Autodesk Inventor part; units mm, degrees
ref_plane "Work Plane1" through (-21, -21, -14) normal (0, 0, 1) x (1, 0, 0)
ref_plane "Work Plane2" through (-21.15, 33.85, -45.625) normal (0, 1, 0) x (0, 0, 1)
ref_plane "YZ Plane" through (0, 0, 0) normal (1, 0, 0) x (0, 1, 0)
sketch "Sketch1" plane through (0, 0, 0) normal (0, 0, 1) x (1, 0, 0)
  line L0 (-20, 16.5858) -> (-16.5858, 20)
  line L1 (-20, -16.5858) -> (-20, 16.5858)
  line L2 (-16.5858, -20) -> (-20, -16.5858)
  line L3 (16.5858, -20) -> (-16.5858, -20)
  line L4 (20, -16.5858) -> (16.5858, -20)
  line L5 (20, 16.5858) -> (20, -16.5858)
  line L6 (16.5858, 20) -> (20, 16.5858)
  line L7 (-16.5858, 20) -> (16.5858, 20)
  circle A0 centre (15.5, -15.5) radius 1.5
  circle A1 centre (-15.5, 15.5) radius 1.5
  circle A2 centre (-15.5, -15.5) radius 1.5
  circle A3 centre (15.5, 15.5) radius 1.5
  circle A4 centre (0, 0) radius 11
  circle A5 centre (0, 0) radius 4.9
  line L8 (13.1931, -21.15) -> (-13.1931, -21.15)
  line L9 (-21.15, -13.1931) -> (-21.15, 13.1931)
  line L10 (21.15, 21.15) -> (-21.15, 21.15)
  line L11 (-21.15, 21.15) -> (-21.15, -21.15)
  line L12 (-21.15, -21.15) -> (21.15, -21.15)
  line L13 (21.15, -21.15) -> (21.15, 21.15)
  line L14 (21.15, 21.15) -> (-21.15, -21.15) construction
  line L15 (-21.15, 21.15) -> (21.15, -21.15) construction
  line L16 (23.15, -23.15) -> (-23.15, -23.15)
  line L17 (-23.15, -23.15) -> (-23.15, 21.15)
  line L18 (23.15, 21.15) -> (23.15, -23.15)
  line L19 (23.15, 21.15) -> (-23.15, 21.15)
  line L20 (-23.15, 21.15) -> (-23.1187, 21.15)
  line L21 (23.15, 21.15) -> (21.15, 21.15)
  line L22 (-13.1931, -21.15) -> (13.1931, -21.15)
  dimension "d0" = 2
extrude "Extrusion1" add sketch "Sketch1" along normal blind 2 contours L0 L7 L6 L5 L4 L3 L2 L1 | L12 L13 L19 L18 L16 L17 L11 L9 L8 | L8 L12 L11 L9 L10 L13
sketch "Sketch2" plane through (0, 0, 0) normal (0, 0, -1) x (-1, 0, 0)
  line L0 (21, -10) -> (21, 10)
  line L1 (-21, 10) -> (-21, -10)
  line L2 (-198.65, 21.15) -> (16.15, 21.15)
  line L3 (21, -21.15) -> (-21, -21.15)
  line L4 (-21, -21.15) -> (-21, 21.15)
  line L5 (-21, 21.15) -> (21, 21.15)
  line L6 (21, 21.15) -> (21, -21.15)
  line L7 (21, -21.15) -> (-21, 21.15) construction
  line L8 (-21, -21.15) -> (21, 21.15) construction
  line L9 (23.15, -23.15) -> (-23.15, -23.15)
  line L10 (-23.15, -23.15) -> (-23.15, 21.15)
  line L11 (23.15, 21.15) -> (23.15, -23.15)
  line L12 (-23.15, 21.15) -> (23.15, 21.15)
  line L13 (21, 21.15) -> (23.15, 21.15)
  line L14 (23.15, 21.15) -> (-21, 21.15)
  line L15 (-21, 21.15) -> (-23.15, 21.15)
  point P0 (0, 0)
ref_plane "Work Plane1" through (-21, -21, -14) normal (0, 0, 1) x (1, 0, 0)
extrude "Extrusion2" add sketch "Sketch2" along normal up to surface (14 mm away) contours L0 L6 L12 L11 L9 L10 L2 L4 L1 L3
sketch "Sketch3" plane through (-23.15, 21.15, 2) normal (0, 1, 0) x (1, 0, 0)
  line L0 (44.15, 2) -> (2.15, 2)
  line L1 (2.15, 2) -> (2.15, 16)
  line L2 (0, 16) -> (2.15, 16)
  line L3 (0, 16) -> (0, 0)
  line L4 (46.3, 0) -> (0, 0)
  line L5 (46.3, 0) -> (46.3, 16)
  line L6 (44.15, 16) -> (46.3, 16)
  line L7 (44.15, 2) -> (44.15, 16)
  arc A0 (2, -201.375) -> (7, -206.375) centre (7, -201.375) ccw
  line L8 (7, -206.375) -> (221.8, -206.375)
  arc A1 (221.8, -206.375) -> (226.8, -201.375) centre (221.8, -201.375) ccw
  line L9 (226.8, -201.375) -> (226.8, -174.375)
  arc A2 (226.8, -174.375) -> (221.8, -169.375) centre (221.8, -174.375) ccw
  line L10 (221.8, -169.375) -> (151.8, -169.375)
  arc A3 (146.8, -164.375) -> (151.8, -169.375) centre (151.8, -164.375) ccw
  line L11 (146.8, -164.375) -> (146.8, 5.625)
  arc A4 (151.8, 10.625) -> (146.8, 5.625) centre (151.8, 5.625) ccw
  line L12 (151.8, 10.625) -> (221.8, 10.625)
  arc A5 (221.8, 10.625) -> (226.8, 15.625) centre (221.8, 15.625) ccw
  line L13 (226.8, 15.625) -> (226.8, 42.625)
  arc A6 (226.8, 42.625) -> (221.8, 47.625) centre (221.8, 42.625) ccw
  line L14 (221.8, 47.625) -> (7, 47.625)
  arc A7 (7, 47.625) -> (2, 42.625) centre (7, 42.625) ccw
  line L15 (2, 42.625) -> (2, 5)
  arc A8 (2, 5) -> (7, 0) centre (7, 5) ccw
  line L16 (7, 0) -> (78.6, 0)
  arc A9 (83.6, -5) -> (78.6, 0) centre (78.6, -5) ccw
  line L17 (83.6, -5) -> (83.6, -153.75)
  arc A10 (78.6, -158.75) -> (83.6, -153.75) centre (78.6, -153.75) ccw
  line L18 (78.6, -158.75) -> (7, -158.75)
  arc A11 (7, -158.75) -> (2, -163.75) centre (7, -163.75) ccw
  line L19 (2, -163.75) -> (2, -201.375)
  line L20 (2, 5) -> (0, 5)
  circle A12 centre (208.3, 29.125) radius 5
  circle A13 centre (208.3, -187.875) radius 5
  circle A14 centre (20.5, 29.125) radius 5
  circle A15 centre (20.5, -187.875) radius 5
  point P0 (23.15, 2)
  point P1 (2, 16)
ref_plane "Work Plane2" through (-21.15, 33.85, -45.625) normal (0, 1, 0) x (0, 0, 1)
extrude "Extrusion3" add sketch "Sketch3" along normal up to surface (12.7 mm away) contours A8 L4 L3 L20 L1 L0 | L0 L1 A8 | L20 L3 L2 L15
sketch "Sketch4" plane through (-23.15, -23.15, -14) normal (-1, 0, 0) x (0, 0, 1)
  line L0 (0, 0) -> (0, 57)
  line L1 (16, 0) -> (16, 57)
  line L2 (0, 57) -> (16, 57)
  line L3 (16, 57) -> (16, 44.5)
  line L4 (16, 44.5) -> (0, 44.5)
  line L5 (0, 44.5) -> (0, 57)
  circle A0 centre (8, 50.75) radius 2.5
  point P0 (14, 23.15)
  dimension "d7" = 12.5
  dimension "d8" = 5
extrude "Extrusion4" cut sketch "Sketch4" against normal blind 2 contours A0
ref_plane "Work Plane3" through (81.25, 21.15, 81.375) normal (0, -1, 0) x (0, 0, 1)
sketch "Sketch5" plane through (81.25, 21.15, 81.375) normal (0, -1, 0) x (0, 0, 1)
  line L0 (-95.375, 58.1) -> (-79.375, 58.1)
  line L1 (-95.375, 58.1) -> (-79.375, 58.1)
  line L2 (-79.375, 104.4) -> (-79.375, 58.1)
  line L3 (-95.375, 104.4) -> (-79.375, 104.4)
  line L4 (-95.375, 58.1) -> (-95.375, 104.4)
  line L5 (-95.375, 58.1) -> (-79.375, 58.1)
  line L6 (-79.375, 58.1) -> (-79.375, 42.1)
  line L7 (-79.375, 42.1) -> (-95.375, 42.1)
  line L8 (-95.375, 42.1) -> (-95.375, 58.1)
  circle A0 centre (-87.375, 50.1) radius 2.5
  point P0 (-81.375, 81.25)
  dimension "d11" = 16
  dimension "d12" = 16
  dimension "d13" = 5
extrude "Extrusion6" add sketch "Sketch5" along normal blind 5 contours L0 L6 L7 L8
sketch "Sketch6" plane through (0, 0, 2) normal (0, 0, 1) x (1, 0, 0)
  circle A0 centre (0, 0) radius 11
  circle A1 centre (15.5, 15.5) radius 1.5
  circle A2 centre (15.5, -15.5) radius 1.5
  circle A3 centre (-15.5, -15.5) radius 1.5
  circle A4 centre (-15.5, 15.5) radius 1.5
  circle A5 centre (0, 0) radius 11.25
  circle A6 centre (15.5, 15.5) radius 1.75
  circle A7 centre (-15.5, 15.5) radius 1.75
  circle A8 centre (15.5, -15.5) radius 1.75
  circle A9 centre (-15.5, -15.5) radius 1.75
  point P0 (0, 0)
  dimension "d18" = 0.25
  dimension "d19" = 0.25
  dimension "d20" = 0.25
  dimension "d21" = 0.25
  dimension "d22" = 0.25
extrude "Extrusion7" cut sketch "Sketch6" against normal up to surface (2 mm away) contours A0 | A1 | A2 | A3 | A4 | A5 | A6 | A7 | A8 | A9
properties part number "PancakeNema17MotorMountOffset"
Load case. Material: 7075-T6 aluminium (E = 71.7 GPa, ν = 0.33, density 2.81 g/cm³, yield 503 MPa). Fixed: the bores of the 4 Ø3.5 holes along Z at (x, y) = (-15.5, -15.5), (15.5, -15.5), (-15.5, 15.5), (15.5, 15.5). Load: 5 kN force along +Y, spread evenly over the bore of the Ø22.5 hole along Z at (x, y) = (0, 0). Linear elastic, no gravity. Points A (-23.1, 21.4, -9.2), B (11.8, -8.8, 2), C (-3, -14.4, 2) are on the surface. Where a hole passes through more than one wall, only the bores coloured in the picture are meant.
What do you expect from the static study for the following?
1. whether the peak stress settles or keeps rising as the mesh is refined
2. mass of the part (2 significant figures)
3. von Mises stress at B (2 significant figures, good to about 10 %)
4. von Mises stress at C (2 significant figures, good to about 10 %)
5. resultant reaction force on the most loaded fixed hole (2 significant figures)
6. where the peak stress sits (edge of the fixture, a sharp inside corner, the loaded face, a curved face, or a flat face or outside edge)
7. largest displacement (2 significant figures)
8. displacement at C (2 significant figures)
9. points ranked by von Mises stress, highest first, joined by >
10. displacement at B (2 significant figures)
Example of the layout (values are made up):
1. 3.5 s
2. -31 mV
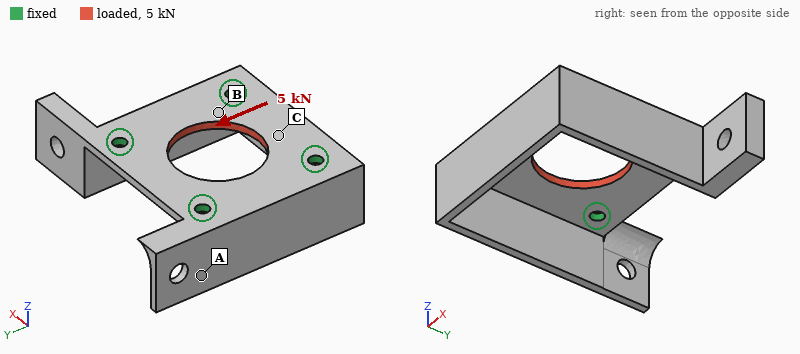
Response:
1. keeps rising
2. 24 g
3. 52 MPa
4. 31 MPa
5. 1.3 kN
6. edge of the fixture
7. 21 µm
8. 14 µm
9. B > C > A
10. 6.3 µm
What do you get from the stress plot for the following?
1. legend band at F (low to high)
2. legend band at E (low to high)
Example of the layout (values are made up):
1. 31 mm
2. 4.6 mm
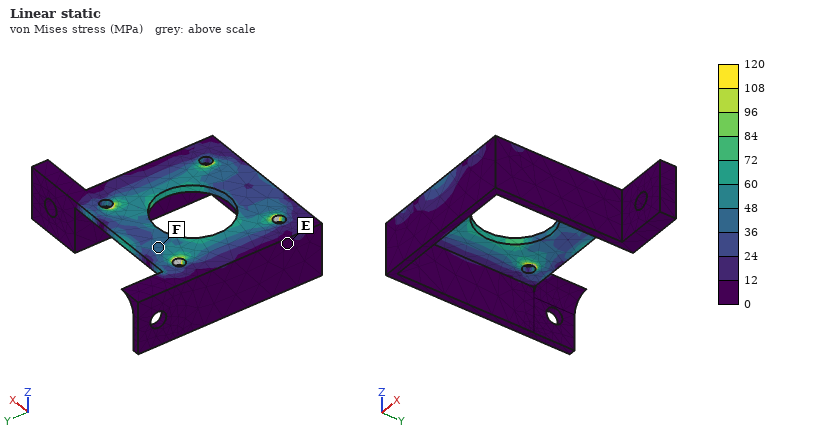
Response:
1. 36 to 48 MPa
2. 0 to 12 MPa
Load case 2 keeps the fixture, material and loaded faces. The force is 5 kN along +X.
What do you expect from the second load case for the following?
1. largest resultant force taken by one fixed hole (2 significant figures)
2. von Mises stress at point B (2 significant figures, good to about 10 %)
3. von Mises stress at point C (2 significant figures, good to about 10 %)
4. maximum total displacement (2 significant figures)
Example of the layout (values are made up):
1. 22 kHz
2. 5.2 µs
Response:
1. 1.3 kN
2. 39 MPa
3. 43 MPa
4. 17 µm
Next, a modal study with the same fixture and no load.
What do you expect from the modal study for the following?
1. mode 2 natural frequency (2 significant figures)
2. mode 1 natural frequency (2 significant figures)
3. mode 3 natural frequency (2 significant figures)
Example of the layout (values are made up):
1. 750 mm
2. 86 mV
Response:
1. 3900 Hz
2. 2100 Hz
3. 5700 Hz
